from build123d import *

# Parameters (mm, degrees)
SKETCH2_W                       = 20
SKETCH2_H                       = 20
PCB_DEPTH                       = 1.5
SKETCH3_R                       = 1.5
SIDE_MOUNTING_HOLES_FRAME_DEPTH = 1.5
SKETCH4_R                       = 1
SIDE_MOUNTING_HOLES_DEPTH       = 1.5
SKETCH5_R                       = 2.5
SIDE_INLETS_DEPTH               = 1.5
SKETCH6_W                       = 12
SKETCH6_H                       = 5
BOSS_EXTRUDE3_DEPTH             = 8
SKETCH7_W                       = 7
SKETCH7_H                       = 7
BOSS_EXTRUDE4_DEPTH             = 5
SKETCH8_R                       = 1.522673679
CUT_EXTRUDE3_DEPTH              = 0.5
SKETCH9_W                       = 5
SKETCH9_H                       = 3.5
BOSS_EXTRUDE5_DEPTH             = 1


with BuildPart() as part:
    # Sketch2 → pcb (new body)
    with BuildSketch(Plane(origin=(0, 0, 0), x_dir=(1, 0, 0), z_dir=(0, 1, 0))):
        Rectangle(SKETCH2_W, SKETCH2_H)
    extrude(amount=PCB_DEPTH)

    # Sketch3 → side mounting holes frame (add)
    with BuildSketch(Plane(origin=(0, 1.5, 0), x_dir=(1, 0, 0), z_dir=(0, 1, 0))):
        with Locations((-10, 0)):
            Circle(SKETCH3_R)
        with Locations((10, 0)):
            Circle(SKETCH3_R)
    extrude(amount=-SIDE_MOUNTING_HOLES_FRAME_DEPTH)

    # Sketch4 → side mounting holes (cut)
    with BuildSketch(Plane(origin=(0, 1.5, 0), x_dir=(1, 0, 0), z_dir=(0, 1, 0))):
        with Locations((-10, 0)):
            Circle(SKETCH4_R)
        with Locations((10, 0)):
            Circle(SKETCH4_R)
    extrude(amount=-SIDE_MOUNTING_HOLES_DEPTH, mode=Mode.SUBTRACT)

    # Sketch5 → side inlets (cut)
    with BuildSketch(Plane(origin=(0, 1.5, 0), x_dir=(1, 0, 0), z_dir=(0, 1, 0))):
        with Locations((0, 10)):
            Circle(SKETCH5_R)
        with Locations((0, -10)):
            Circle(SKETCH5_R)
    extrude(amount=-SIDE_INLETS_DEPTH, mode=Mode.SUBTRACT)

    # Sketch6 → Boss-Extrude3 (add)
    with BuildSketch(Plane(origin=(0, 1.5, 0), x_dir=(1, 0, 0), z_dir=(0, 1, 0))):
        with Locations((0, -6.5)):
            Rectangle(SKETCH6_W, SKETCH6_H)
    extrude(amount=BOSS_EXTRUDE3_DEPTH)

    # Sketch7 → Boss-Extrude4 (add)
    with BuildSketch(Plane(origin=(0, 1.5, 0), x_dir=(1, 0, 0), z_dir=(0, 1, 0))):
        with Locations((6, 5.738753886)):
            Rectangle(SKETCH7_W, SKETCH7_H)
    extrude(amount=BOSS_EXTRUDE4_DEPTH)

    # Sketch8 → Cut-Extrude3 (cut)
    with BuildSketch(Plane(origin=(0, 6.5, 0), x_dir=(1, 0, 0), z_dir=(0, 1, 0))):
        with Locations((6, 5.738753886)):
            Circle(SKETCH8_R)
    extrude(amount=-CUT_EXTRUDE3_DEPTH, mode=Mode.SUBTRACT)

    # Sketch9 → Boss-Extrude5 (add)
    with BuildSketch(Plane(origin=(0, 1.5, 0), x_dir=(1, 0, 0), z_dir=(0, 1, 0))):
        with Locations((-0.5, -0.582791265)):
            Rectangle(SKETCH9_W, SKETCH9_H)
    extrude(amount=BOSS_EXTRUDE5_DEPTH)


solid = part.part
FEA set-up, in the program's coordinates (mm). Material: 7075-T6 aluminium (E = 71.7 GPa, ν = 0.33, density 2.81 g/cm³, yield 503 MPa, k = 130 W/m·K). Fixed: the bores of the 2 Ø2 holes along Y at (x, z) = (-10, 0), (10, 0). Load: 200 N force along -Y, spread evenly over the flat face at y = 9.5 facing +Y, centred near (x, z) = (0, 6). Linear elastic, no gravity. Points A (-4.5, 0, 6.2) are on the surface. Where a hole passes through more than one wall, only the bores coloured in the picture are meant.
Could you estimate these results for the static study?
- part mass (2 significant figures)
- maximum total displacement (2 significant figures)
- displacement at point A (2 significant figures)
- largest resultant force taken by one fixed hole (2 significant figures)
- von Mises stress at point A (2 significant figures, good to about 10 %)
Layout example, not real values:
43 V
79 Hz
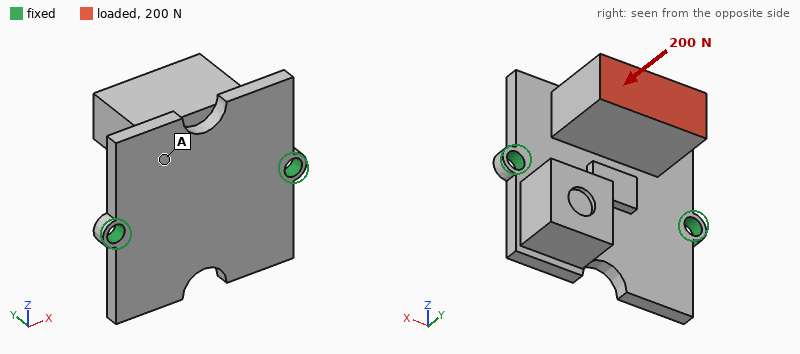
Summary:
3.7 g
0.17 mm
0.078 mm
100 N
40 MPa
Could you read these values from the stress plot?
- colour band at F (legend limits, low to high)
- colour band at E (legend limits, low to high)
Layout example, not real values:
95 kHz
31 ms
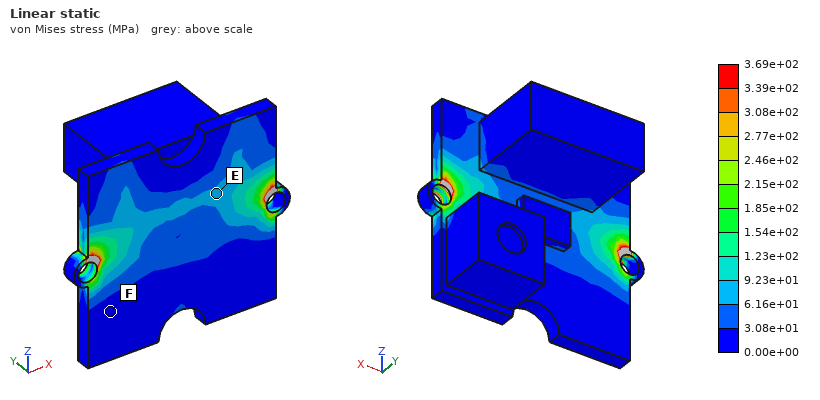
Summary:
0.00e+00 to 3.08e+01 MPa
6.16e+01 to 9.23e+01 MPa
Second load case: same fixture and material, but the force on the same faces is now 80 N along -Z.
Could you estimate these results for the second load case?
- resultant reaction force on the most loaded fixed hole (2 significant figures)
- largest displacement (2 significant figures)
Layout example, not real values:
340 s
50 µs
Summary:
40 N
0.12 mm
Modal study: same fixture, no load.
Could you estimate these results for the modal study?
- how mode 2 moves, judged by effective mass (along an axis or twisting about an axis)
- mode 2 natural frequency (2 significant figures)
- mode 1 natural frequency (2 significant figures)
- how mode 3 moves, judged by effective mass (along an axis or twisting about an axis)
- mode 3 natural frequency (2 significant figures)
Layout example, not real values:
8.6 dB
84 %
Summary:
along Y
7400 Hz
4100 Hz
along Y
13 kHz
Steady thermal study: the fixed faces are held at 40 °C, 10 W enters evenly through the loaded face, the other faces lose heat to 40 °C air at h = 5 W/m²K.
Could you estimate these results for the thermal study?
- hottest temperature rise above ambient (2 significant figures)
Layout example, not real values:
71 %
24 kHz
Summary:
35 K
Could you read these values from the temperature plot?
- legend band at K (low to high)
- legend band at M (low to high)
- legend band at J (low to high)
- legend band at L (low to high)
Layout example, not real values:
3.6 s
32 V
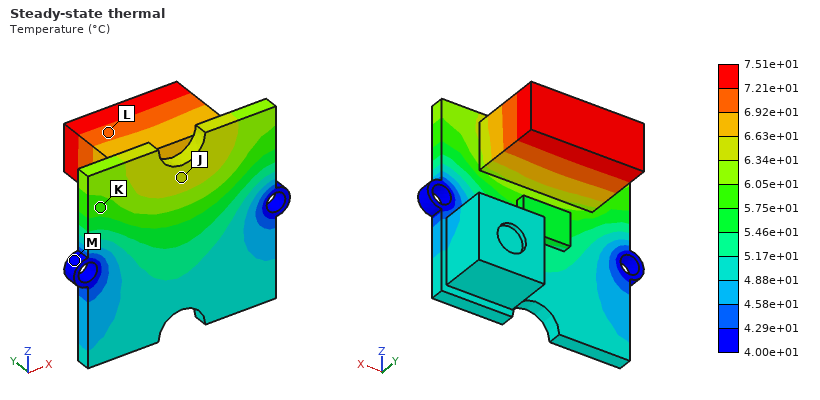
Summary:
5.75e+01 to 6.05e+01 °C
4.00e+01 to 4.29e+01 °C
6.34e+01 to 6.63e+01 °C
6.92e+01 to 7.21e+01 °C
